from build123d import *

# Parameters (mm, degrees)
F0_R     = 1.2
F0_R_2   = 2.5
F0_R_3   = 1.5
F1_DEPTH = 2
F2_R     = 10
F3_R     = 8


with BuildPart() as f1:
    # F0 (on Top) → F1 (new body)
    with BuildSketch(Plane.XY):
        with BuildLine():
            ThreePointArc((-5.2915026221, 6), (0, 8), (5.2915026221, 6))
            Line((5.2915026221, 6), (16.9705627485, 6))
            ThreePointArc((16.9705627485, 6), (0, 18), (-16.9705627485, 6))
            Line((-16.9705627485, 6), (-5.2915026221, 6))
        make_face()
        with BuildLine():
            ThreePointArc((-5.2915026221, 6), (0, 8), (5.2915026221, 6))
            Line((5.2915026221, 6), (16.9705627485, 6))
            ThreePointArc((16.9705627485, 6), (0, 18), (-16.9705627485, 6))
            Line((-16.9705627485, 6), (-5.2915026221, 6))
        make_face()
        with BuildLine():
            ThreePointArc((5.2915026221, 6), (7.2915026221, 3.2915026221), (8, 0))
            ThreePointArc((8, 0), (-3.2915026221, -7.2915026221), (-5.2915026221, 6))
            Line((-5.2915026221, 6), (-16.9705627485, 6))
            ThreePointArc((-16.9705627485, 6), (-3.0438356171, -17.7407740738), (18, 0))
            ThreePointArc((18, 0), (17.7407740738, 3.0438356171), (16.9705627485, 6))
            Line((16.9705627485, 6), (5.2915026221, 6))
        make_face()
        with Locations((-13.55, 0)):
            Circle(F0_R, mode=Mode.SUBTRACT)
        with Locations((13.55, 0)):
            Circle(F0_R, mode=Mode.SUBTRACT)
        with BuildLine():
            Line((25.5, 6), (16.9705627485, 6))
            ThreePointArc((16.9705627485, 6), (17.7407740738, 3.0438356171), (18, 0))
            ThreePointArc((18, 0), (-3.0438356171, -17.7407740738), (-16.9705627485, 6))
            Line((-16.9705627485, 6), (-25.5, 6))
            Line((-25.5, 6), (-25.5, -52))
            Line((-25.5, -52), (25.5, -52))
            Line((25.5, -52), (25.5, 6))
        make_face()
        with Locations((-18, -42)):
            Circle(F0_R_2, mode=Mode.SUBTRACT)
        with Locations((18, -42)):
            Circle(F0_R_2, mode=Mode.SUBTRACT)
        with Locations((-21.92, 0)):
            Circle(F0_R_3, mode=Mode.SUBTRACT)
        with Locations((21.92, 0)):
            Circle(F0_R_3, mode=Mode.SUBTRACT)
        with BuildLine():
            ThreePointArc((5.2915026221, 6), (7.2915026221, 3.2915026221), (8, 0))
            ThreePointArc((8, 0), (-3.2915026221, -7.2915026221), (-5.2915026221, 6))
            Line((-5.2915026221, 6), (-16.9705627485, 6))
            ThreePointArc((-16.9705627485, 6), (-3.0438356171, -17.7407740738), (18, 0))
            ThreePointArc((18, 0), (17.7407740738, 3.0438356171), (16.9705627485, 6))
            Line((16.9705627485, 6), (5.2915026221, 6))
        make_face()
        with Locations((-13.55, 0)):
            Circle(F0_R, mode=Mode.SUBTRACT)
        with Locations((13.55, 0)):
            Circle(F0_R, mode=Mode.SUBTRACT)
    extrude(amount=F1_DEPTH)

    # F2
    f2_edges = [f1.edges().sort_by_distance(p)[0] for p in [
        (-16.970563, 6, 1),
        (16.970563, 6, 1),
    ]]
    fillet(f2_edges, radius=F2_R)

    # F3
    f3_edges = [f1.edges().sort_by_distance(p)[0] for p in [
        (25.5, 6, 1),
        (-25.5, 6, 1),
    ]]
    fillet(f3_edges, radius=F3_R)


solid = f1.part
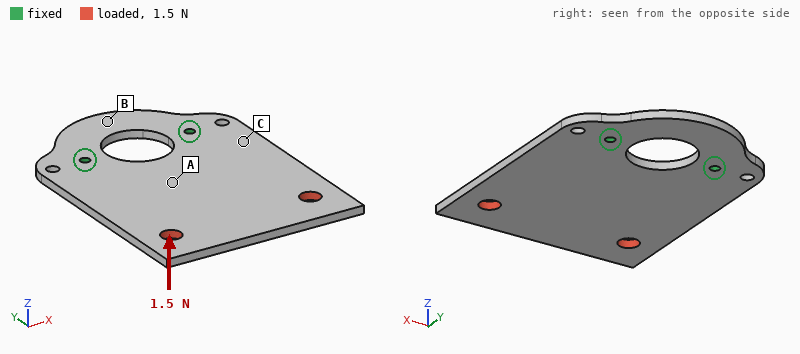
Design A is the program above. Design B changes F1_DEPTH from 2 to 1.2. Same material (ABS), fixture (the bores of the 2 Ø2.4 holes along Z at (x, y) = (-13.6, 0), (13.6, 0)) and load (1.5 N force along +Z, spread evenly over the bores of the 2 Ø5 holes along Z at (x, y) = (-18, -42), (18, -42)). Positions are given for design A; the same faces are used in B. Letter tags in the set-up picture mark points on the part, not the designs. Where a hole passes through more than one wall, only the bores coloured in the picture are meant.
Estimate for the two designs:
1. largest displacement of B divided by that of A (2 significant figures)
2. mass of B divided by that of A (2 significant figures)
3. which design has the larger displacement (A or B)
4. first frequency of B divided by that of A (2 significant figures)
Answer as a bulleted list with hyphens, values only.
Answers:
- 4.5
- 0.60
- B
- 0.61
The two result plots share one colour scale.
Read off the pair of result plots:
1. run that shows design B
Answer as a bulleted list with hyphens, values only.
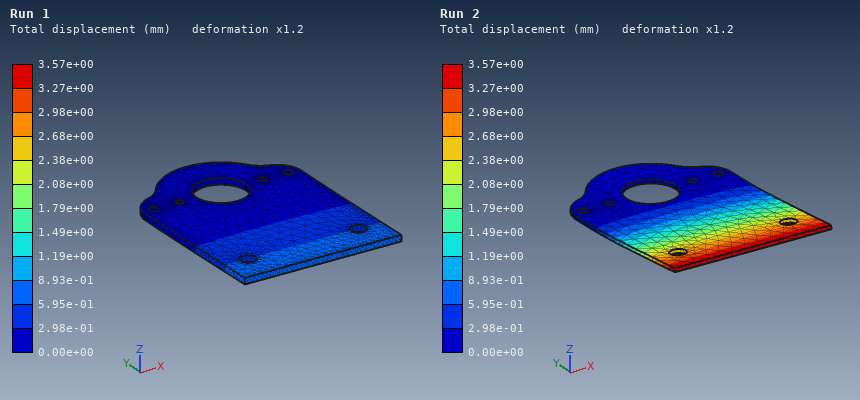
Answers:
- Run 2
